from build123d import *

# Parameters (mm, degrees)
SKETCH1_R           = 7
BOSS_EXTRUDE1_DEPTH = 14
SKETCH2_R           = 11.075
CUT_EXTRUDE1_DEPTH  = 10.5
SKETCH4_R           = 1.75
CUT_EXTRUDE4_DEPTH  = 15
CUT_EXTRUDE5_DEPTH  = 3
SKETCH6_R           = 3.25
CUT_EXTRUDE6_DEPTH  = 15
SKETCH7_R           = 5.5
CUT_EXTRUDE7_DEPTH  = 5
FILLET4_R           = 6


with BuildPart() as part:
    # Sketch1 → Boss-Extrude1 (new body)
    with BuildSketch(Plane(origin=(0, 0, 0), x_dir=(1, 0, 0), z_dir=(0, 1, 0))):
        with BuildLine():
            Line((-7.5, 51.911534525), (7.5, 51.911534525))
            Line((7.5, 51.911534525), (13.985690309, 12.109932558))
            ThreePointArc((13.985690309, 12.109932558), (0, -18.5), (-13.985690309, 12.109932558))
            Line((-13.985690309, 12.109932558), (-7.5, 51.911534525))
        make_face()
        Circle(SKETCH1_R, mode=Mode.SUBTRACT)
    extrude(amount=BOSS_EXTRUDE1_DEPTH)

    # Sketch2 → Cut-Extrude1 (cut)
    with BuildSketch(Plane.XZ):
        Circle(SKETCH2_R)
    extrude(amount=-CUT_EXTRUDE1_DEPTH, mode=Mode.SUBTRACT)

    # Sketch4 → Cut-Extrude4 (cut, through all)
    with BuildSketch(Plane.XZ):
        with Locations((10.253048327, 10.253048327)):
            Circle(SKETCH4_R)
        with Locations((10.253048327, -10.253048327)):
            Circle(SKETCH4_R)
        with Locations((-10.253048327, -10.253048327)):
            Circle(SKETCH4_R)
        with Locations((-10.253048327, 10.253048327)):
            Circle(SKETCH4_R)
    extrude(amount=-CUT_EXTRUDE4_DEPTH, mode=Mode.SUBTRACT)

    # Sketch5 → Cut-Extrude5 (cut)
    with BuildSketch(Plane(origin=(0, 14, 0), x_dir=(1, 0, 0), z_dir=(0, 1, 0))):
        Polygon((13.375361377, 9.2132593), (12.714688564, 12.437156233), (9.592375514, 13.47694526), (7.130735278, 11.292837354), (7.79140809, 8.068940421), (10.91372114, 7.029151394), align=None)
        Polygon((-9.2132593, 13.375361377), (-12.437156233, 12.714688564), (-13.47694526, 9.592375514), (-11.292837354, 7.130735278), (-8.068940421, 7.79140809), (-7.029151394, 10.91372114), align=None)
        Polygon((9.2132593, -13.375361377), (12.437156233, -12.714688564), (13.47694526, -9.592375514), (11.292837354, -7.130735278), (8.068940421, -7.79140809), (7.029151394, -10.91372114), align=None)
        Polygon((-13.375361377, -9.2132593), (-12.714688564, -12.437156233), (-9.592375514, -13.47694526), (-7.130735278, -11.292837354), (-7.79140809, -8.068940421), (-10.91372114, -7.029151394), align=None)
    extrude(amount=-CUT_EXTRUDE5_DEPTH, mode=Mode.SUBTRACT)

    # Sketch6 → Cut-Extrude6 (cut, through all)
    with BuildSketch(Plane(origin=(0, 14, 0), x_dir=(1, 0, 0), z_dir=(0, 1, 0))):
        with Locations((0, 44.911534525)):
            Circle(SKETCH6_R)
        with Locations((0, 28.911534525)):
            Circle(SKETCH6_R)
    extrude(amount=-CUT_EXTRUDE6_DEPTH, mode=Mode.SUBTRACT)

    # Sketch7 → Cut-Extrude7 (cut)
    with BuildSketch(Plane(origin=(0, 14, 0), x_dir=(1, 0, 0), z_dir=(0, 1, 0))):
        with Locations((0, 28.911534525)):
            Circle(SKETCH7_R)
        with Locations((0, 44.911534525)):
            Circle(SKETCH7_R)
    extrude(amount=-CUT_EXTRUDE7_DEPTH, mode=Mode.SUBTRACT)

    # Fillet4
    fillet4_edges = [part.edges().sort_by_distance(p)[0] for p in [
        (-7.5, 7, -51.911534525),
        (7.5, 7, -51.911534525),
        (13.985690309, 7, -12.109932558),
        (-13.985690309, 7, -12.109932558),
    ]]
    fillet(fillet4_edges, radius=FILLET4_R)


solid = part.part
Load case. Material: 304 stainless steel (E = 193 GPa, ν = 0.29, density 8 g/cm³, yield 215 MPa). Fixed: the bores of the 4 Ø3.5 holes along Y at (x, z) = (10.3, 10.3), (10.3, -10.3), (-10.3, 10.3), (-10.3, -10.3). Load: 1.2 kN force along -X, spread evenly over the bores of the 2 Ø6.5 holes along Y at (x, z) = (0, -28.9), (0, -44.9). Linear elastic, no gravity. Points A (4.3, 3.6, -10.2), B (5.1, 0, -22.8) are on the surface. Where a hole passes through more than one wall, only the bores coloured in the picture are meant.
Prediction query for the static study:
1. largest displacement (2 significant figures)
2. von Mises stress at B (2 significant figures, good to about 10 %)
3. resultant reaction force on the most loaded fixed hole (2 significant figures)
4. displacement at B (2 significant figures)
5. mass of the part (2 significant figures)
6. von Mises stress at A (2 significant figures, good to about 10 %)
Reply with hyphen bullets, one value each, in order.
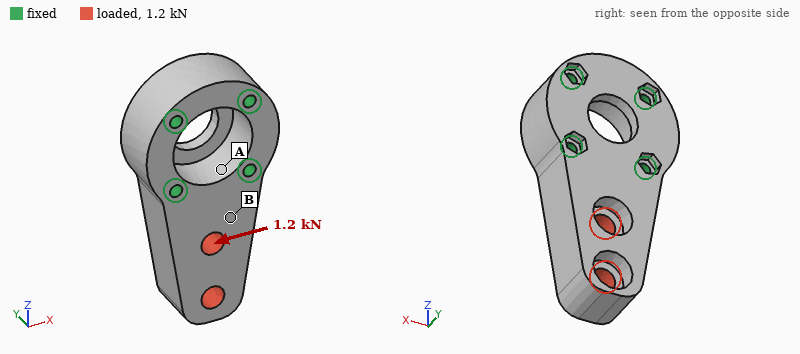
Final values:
- 6.7 µm
- 9.3 MPa
- 1.5 kN
- 1.3 µm
- 150 g
- 3.8 MPa
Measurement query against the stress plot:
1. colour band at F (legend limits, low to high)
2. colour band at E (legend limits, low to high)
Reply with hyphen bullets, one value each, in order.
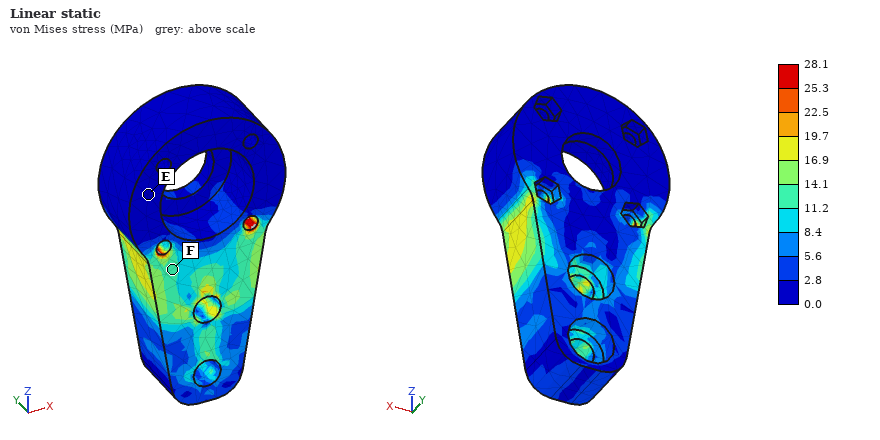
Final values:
- 11.2 to 14.1 MPa
- 0.0 to 2.8 MPa
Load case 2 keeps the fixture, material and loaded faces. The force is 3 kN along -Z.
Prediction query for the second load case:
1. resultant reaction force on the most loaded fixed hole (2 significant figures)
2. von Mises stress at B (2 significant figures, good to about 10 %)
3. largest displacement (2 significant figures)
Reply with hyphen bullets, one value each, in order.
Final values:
- 1.5 kN
- 19 MPa
- 7.2 µm
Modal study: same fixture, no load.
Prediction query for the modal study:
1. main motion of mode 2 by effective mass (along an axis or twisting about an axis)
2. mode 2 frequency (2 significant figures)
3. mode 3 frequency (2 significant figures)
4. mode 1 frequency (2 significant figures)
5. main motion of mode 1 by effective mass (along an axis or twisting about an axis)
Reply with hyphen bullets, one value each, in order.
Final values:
- along X
- 12 kHz
- 18 kHz
- 6300 Hz
- along Y
